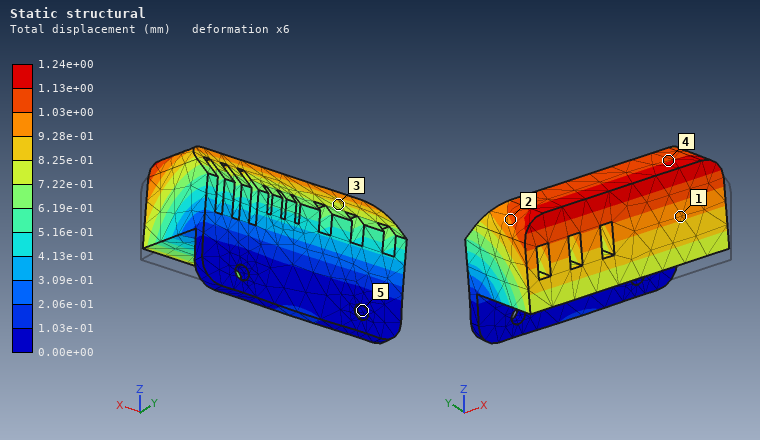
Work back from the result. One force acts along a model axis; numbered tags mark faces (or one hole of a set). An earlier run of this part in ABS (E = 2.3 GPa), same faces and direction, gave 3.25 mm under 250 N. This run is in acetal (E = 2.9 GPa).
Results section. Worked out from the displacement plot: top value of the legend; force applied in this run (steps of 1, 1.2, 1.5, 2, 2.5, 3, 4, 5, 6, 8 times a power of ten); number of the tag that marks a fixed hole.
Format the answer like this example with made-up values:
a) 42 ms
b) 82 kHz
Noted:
a) 1.24e+00 mm
b) 120 N
c) 5
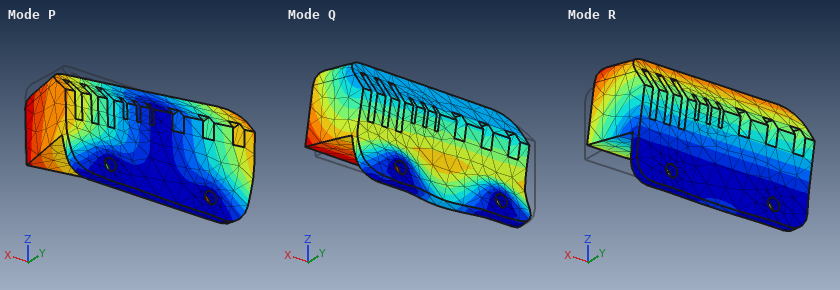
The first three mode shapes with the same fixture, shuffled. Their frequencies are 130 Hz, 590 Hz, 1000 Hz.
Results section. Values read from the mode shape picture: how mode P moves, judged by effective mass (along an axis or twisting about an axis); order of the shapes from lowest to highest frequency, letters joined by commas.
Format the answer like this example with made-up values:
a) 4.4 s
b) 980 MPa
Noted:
a) along X
b) R, P, Q
